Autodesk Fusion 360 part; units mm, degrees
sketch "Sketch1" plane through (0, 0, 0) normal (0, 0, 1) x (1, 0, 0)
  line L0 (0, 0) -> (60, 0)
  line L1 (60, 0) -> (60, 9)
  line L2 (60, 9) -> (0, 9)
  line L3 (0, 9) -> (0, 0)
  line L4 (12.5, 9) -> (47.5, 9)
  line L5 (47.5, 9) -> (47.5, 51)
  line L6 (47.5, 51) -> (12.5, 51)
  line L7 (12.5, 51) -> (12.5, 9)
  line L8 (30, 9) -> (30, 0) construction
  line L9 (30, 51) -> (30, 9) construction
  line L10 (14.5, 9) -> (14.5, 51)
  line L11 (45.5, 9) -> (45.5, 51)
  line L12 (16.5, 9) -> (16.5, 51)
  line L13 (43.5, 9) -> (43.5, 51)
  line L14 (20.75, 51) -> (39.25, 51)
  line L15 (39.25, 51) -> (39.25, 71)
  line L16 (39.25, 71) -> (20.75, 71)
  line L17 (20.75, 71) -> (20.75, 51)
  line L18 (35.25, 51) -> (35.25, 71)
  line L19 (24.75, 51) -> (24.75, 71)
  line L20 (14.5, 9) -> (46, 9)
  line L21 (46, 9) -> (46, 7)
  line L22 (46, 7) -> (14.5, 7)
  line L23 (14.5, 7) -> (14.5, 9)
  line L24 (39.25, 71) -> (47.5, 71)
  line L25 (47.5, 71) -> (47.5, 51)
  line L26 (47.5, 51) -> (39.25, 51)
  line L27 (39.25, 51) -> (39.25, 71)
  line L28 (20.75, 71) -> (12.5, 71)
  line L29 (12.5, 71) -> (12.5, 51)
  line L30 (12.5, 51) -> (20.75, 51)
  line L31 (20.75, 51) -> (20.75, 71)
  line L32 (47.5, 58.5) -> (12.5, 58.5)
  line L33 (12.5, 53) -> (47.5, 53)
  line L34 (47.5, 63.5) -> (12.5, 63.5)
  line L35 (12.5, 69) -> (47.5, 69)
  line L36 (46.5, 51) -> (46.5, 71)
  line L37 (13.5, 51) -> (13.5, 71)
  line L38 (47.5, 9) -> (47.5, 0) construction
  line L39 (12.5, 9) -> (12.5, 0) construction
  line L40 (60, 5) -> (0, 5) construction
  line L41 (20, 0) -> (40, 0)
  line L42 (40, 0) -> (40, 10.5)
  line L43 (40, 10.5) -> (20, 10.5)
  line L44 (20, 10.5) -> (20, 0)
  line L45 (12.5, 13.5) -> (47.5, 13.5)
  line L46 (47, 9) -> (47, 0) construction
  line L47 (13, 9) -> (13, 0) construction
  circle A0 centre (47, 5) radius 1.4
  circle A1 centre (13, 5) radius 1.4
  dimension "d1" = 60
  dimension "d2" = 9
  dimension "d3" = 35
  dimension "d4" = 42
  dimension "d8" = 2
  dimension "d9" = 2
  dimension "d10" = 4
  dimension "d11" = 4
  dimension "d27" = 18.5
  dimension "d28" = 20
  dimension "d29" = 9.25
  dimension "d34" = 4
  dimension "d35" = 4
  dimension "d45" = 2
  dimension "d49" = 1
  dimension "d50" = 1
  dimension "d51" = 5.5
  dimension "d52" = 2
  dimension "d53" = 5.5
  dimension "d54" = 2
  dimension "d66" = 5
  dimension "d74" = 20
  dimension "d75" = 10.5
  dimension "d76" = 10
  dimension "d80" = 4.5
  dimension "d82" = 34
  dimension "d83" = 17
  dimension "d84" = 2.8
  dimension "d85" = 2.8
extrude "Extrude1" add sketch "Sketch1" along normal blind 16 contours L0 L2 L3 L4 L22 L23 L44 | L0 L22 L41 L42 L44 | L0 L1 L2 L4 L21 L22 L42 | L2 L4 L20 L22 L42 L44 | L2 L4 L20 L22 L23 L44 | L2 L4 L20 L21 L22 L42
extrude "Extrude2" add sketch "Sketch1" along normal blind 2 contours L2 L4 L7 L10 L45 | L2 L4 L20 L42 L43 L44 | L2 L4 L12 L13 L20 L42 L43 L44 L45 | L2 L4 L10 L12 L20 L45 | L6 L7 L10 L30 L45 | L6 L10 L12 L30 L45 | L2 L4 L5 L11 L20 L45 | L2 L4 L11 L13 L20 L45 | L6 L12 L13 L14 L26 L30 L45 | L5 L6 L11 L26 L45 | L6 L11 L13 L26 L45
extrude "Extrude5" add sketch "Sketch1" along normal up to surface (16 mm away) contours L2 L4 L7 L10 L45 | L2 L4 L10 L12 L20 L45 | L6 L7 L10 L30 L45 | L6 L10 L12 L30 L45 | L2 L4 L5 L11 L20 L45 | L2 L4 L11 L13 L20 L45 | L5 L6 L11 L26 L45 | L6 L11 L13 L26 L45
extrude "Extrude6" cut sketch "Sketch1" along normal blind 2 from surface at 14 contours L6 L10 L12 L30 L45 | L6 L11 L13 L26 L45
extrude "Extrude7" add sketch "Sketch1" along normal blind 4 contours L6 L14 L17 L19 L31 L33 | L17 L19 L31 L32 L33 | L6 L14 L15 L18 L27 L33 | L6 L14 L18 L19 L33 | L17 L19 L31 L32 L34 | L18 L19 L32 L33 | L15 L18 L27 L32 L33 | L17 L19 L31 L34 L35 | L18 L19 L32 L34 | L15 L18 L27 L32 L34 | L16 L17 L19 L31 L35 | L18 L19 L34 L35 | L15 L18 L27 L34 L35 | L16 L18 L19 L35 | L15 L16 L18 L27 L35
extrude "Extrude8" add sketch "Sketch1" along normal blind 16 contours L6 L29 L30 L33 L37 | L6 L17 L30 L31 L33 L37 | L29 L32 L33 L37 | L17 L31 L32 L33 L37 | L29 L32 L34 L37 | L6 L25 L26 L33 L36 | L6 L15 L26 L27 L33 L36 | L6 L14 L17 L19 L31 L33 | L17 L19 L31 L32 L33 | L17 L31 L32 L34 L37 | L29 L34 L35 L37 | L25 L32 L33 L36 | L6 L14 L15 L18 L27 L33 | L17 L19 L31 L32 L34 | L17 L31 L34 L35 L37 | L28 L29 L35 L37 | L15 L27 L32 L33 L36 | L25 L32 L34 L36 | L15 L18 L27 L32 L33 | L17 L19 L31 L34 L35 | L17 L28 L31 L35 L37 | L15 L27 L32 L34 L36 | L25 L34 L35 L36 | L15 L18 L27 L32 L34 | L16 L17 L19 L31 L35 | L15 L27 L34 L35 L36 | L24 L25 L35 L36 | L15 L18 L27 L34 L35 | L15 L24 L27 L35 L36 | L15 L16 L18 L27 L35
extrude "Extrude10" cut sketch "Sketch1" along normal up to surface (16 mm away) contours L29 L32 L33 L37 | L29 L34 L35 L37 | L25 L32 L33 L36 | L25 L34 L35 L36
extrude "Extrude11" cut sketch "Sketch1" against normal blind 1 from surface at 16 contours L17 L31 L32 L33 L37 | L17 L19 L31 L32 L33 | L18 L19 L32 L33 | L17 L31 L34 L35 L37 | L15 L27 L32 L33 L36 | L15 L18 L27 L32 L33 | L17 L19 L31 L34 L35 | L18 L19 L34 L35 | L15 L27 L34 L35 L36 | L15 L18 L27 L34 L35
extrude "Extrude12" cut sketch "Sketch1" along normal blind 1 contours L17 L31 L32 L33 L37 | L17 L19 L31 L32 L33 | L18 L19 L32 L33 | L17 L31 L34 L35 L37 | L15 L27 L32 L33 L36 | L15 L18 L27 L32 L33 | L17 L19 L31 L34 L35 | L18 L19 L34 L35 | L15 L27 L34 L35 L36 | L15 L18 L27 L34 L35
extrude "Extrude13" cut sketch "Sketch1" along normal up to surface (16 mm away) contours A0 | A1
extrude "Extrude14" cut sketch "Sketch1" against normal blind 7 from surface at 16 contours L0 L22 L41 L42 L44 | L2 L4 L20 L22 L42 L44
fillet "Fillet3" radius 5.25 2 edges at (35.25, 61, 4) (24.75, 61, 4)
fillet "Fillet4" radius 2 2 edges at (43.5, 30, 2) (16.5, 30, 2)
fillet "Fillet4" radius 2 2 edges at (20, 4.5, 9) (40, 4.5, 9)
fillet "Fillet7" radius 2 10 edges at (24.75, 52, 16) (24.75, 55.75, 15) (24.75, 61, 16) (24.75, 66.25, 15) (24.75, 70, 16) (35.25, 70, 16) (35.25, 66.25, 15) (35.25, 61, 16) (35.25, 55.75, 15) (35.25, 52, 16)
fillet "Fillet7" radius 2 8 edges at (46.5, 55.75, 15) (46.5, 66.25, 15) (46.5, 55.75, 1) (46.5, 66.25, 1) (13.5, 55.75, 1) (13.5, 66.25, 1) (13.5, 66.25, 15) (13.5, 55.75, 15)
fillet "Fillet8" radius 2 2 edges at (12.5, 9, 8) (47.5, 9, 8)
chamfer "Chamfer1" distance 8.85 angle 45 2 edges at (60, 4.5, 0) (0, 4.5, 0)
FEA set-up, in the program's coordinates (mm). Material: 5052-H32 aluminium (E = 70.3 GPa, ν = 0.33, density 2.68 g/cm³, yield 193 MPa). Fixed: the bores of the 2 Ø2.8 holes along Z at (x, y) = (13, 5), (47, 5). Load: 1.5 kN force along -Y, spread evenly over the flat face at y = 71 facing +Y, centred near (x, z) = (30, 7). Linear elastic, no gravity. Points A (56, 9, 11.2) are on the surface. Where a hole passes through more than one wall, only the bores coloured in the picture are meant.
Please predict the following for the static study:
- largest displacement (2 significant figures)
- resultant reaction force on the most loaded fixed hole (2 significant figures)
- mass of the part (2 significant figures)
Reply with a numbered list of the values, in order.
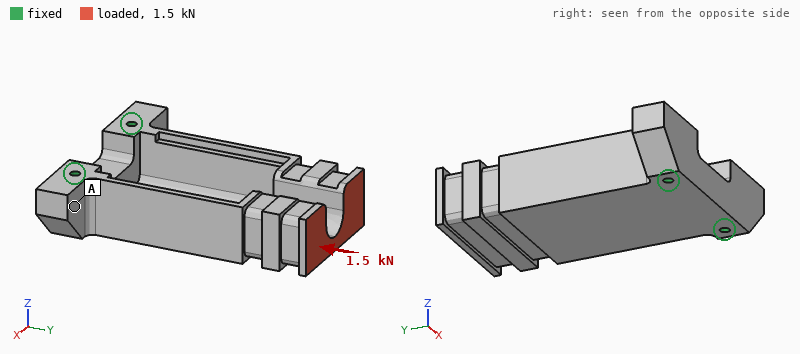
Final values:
1. 22 µm
2. 750 N
3. 59 g
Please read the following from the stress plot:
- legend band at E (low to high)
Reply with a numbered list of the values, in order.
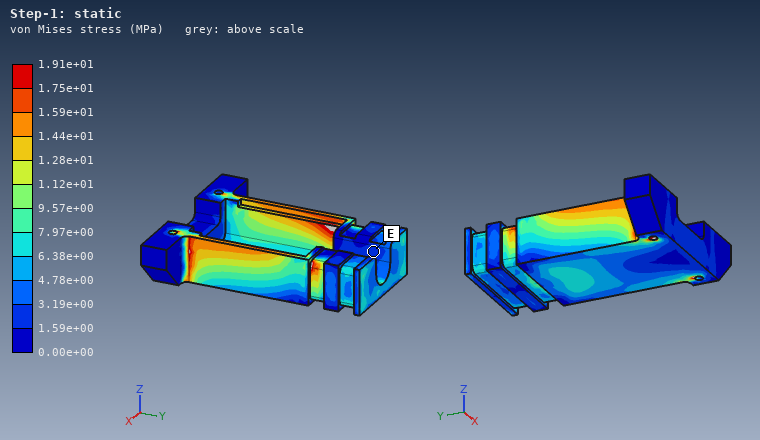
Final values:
1. 1.59e+00 to 3.19e+00 MPa
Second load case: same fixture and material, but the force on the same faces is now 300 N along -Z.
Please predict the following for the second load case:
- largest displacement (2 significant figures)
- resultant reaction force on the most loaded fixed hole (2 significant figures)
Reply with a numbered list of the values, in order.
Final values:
1. 0.12 mm
2. 200 N
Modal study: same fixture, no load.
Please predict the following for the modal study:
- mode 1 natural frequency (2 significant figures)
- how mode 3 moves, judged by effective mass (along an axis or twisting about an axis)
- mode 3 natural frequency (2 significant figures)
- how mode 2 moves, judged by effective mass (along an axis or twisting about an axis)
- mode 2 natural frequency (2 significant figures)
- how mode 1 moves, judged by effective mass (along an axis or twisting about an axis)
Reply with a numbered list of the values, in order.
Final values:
1. 2000 Hz
2. along X
3. 6200 Hz
4. along X
5. 2600 Hz
6. along Z
